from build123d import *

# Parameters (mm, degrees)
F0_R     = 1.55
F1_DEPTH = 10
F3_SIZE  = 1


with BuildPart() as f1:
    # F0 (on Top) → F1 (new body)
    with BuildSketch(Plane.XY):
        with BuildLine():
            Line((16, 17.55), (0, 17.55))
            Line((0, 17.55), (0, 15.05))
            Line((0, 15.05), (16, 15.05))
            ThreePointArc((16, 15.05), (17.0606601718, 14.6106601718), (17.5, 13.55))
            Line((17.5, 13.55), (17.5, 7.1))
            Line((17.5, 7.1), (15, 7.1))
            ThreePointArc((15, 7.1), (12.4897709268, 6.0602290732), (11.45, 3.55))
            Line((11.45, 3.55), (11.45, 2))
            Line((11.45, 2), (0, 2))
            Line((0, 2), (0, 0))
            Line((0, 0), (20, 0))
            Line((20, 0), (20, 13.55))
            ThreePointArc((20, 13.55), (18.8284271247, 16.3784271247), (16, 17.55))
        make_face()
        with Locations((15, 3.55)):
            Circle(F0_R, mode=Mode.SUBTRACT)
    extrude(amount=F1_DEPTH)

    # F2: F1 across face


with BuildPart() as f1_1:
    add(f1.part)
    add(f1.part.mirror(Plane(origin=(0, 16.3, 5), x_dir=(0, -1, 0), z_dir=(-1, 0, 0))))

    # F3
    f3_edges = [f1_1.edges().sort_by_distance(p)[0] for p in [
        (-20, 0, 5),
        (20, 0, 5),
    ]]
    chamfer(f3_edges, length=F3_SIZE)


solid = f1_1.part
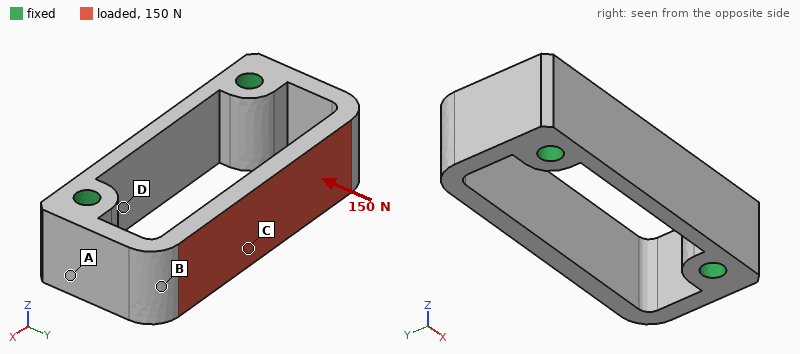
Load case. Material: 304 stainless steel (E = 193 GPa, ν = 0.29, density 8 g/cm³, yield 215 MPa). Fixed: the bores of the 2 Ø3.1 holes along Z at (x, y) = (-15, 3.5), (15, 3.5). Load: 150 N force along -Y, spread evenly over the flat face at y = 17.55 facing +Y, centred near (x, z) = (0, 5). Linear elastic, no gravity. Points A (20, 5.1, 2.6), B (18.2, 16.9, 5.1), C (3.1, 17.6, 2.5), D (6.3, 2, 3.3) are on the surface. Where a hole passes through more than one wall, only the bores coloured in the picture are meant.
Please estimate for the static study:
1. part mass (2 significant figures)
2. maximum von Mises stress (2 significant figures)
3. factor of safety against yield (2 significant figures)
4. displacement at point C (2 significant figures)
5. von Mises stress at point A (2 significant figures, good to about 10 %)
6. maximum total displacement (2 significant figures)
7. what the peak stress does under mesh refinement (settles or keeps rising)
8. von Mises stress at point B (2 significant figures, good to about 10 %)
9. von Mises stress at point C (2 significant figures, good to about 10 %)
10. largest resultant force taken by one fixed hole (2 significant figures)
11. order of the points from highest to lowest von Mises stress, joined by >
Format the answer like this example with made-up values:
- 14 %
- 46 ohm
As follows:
- 22 g
- 55 MPa
- 3.9
- 12 µm
- 8.3 MPa
- 13 µm
- settles
- 21 MPa
- 30 MPa
- 100 N
- C > B > A > D
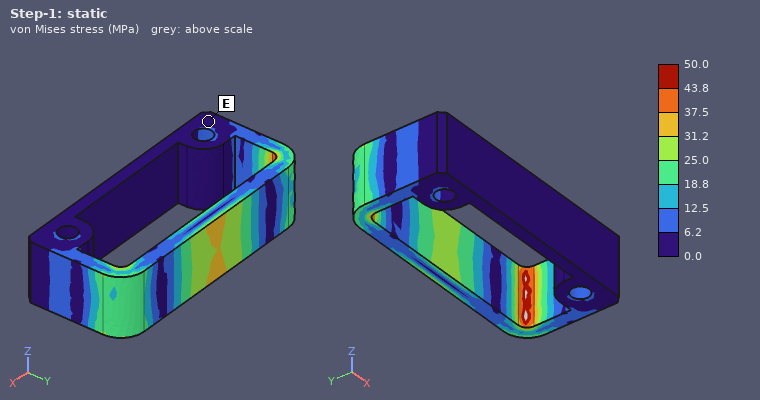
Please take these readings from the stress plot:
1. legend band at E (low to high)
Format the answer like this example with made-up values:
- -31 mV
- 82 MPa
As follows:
- 0.0 to 6.2 MPa
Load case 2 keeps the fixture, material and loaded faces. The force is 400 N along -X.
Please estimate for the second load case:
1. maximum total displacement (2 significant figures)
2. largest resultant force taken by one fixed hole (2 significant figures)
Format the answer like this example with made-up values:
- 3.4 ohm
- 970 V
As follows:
- 18 µm
- 210 N
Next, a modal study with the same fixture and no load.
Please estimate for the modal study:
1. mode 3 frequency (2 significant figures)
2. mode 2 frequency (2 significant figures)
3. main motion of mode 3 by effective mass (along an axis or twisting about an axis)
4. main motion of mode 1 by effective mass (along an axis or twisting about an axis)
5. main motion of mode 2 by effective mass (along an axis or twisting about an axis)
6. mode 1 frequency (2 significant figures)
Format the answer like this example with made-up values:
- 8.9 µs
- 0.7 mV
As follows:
- 11 kHz
- 8300 Hz
- along Z
- along Y
- along X
- 7700 Hz
